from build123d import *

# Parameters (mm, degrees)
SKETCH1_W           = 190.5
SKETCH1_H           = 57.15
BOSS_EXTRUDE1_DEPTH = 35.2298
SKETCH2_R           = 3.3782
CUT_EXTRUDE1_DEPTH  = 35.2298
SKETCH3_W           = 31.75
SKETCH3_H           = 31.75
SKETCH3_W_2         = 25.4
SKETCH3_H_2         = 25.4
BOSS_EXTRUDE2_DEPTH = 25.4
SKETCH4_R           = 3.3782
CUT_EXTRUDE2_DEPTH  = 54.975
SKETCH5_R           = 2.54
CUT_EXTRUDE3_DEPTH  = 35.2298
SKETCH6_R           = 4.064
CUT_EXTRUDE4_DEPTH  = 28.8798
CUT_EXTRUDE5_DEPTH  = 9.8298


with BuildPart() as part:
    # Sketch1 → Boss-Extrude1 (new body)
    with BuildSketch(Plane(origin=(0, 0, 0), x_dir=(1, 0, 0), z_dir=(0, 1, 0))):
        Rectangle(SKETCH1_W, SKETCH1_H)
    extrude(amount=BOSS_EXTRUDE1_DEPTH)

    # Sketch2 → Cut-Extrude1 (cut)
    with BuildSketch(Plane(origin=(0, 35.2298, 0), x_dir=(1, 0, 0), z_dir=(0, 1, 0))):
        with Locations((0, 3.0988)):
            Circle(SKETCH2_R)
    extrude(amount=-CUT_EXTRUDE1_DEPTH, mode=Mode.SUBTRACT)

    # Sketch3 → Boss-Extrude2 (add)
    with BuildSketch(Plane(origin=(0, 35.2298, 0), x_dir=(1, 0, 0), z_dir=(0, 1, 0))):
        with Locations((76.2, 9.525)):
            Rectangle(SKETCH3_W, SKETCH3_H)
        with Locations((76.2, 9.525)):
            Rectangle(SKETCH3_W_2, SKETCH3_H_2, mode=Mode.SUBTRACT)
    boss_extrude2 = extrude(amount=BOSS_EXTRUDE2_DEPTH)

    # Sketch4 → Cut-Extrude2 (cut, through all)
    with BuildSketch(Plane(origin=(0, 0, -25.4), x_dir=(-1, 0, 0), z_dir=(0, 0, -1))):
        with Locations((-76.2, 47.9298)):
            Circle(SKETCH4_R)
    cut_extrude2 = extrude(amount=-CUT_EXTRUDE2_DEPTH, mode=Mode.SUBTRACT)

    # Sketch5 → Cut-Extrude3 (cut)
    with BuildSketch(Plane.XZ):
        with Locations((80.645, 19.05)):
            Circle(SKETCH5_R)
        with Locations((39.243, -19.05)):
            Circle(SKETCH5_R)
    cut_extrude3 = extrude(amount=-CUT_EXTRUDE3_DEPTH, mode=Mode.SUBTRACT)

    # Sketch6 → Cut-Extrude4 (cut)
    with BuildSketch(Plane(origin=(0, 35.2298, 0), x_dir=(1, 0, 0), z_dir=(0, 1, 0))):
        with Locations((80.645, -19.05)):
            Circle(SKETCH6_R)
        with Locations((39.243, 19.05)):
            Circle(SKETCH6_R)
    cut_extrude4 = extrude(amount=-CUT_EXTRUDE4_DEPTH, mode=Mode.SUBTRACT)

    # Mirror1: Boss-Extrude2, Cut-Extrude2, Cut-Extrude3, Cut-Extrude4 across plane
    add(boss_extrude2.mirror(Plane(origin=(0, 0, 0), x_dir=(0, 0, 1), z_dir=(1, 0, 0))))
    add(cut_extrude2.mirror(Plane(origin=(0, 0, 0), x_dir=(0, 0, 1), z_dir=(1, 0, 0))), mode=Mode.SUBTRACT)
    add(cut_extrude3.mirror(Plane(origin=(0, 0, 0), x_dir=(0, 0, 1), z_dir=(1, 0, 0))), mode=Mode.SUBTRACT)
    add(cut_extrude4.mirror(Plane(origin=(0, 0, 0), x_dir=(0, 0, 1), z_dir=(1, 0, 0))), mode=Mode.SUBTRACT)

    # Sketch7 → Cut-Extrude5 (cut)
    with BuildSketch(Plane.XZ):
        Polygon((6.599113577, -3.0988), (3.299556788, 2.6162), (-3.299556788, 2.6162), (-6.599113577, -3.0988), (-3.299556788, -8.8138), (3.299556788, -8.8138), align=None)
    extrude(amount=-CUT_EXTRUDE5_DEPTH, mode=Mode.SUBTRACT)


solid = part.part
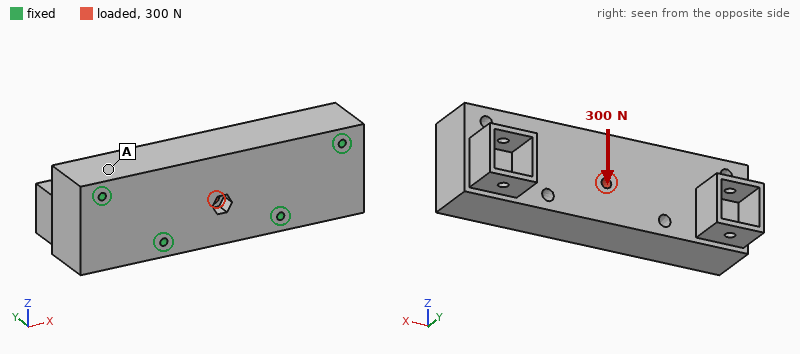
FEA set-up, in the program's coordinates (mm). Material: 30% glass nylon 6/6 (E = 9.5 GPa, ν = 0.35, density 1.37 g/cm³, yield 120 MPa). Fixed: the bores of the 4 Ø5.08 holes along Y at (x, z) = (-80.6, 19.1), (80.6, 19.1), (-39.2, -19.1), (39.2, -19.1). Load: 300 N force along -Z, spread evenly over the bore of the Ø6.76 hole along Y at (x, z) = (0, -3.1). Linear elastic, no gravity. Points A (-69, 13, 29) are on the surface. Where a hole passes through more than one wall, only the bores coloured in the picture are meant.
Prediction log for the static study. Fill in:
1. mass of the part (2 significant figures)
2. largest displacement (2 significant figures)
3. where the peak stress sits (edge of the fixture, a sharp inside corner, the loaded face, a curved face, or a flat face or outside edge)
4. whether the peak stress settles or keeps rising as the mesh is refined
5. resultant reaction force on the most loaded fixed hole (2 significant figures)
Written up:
540 g
7.6 µm
edge of the fixture
keeps rising
140 N
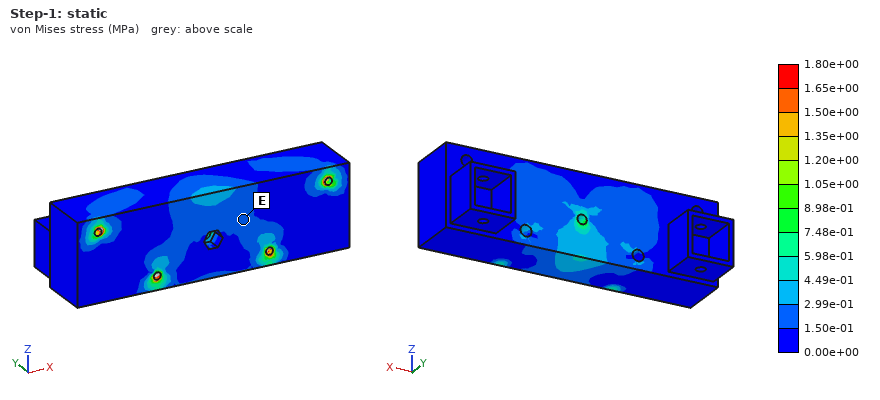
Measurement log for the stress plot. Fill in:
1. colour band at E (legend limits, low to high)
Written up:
1.50e-01 to 2.99e-01 MPa
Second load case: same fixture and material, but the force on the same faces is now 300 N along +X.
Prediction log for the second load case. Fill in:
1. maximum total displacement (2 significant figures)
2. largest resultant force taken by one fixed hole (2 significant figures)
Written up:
1.9 µm
92 N
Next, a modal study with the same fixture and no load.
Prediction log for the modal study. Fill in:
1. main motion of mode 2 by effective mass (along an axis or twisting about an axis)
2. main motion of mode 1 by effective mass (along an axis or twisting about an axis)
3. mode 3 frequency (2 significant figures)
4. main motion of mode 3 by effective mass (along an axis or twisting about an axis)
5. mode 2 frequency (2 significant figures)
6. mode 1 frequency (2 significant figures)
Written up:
along X
along Z
3400 Hz
along Y
2600 Hz
1700 Hz
